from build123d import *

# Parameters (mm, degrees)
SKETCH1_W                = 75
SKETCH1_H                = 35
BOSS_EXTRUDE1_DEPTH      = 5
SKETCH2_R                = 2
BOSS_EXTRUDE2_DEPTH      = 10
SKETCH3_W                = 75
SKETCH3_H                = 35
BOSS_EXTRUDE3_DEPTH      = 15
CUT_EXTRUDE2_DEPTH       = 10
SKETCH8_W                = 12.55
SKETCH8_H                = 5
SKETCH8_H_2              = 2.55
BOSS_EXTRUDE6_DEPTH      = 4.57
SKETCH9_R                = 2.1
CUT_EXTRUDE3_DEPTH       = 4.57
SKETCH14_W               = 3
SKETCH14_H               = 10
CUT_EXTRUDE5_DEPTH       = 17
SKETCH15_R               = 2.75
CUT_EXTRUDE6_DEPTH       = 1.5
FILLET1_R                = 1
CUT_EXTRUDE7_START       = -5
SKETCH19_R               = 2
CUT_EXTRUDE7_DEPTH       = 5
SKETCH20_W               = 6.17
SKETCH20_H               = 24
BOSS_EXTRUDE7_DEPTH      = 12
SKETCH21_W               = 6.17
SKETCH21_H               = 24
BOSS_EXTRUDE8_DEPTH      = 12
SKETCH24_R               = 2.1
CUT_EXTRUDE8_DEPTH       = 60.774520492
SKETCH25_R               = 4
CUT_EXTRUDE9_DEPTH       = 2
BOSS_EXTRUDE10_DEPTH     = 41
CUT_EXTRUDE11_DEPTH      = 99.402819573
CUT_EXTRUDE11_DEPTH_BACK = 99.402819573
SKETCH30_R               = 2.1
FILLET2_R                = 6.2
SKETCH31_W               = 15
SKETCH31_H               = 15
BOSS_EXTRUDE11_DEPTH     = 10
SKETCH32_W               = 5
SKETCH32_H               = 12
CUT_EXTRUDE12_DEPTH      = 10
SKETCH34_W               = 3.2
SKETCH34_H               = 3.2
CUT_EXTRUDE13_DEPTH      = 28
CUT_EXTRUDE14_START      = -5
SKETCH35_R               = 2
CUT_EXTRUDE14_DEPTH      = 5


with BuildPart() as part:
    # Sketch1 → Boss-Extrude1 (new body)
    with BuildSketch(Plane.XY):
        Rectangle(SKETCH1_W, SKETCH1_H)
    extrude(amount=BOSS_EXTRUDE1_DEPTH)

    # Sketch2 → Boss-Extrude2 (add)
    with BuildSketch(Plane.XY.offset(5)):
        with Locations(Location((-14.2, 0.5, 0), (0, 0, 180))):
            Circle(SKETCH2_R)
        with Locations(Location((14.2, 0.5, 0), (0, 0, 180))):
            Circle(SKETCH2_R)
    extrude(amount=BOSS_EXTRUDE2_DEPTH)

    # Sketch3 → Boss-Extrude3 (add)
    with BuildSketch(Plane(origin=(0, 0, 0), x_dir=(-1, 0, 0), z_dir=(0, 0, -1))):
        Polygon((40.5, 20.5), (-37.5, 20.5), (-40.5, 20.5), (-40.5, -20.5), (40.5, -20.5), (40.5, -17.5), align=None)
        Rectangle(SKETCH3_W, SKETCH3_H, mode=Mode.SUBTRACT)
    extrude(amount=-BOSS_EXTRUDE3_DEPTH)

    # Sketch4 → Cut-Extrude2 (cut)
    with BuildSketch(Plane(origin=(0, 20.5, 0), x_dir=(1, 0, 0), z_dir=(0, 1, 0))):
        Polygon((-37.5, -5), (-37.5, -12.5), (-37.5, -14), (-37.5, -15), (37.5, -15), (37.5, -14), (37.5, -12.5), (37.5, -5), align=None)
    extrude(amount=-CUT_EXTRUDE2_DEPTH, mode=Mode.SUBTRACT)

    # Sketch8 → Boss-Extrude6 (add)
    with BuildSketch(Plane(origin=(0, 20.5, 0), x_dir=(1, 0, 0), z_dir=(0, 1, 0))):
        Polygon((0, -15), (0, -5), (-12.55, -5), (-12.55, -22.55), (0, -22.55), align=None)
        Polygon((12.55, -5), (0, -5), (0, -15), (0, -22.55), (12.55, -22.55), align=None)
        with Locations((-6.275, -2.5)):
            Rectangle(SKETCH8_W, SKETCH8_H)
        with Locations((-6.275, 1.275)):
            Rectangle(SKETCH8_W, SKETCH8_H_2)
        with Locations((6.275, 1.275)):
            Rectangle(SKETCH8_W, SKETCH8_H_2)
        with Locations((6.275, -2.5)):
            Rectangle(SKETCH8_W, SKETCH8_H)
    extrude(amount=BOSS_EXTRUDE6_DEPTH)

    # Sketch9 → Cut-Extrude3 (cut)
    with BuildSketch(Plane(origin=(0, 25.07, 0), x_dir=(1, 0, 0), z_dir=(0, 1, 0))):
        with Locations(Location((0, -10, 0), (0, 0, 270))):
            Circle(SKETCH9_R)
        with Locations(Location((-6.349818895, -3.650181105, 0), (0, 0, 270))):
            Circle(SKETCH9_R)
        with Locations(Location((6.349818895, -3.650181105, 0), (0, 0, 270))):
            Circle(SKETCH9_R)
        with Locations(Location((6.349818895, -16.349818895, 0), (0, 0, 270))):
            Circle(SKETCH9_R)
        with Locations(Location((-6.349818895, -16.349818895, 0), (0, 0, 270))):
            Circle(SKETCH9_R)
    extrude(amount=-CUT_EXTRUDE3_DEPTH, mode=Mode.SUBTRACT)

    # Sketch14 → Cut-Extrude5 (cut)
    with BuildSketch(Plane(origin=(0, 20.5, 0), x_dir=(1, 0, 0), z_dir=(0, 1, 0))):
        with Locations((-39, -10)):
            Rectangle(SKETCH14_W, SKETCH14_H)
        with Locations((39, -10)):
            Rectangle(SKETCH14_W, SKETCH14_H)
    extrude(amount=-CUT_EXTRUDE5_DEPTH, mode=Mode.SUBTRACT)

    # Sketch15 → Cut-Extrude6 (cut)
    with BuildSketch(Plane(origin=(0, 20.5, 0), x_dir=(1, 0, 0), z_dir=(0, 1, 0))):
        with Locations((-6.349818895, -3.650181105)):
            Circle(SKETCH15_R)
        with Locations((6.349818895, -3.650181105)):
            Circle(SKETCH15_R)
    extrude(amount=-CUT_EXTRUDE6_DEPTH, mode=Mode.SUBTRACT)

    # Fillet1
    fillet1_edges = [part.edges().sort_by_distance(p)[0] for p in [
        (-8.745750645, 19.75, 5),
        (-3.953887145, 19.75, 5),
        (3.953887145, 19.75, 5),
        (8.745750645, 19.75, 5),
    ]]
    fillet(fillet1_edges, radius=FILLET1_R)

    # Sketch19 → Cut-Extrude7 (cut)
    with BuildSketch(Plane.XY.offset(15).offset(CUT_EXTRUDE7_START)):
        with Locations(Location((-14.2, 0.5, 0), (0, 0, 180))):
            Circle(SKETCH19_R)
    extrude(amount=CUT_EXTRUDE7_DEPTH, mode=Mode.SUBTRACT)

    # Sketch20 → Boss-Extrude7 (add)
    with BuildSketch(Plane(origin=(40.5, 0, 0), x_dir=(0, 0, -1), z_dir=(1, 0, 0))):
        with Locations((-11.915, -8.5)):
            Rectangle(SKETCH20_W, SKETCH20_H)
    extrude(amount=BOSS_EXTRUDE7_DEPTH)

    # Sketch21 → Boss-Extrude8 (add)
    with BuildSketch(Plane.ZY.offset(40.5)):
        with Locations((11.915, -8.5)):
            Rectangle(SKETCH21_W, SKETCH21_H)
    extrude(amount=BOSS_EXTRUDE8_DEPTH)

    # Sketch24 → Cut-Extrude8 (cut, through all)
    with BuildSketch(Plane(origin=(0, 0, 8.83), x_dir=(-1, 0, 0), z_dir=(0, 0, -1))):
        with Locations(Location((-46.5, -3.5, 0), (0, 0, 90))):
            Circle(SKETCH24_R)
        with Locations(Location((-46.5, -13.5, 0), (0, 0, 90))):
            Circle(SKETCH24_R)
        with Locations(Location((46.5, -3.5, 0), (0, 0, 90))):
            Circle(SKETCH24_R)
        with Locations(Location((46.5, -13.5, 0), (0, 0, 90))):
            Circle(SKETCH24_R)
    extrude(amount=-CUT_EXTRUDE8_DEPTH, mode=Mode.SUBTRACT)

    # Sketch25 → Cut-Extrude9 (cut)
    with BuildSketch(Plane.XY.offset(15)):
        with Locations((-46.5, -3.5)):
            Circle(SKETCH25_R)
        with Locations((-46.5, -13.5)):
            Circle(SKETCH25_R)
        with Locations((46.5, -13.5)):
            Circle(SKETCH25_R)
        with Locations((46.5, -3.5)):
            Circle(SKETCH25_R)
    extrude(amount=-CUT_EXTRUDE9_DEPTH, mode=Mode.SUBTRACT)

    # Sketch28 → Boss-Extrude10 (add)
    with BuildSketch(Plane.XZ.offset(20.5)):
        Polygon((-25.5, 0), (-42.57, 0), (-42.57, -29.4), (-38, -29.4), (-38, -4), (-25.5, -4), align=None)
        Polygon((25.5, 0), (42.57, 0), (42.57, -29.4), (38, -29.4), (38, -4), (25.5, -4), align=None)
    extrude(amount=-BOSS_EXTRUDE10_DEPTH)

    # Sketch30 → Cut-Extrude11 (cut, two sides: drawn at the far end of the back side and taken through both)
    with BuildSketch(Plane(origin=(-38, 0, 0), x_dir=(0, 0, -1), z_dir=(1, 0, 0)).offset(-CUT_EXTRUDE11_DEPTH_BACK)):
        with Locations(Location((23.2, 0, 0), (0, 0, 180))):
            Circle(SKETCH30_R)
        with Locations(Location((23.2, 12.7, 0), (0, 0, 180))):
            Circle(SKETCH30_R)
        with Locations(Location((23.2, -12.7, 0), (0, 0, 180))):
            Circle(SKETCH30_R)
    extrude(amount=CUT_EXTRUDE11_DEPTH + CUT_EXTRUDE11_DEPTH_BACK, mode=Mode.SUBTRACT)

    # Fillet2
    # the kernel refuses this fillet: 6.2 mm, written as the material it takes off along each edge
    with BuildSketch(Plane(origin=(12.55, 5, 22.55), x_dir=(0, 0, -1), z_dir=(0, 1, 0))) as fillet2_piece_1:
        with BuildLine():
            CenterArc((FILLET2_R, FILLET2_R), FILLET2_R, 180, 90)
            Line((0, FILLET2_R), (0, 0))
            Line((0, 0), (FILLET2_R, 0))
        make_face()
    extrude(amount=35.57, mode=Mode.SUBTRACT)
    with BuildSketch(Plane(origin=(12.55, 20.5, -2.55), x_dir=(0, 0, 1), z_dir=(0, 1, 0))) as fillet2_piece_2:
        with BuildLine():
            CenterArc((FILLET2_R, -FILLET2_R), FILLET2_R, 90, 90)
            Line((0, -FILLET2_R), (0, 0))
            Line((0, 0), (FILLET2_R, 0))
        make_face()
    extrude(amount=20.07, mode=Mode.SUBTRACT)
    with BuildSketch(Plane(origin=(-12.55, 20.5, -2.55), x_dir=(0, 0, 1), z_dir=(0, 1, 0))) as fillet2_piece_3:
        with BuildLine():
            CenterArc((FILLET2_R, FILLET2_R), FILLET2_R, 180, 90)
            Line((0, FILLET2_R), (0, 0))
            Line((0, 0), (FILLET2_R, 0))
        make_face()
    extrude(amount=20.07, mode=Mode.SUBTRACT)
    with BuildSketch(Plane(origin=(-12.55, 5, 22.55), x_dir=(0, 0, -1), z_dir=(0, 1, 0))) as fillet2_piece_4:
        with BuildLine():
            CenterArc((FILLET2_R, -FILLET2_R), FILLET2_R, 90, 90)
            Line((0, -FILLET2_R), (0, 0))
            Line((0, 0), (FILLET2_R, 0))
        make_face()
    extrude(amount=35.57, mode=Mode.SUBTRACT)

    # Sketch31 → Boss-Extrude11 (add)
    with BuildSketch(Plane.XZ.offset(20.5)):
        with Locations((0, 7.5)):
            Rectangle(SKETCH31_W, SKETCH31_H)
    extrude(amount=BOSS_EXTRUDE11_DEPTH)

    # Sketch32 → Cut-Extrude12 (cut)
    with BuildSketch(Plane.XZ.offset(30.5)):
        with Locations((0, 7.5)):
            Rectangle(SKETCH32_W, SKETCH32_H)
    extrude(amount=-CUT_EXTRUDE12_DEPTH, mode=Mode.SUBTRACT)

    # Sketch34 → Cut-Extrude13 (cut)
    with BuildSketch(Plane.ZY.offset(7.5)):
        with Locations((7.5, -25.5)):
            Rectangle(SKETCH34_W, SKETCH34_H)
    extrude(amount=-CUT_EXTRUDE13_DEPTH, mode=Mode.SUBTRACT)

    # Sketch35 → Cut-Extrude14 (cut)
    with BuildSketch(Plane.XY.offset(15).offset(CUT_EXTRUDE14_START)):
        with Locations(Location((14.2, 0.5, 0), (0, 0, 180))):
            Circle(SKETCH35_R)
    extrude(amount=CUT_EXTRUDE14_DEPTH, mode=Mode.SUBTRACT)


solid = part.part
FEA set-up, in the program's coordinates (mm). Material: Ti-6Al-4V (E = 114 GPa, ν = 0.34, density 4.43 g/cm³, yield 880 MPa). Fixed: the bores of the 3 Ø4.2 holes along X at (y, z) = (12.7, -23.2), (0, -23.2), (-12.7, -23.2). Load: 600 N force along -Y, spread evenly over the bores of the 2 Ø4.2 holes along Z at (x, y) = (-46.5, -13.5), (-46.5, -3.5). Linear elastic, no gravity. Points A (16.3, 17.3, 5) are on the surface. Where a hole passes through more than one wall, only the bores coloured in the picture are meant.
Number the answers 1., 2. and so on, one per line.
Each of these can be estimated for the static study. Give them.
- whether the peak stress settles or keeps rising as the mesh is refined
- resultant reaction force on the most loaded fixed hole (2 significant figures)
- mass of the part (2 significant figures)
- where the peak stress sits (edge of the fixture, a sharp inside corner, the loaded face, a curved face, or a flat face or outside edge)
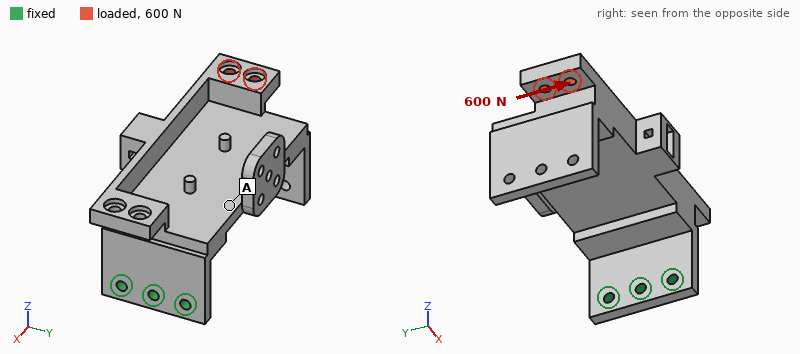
1. keeps rising
2. 1.9 kN
3. 190 g
4. edge of the fixture
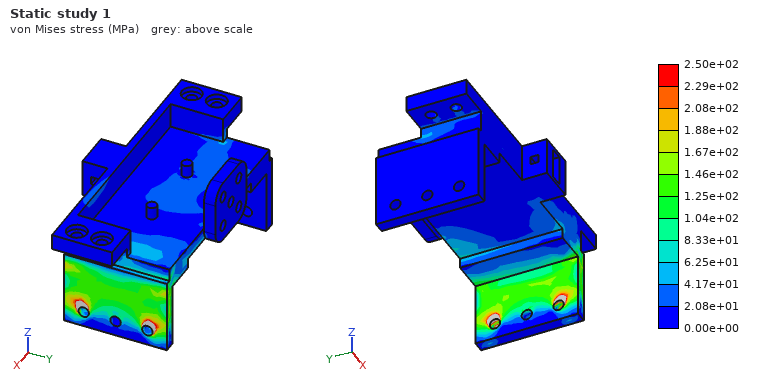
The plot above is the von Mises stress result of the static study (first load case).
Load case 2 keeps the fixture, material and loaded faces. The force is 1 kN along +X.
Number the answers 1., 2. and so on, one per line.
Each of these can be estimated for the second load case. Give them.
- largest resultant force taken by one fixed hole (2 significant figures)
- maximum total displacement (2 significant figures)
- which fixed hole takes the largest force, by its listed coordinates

1. 570 N
2. 1.4 mm
3. (-12.7, -23.2)
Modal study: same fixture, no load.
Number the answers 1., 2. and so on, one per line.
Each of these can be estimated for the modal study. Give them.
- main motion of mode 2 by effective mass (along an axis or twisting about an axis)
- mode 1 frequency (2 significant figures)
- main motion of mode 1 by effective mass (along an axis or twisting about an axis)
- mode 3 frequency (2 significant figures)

1. along Y
2. 280 Hz
3. along Z
4. 1400 Hz
